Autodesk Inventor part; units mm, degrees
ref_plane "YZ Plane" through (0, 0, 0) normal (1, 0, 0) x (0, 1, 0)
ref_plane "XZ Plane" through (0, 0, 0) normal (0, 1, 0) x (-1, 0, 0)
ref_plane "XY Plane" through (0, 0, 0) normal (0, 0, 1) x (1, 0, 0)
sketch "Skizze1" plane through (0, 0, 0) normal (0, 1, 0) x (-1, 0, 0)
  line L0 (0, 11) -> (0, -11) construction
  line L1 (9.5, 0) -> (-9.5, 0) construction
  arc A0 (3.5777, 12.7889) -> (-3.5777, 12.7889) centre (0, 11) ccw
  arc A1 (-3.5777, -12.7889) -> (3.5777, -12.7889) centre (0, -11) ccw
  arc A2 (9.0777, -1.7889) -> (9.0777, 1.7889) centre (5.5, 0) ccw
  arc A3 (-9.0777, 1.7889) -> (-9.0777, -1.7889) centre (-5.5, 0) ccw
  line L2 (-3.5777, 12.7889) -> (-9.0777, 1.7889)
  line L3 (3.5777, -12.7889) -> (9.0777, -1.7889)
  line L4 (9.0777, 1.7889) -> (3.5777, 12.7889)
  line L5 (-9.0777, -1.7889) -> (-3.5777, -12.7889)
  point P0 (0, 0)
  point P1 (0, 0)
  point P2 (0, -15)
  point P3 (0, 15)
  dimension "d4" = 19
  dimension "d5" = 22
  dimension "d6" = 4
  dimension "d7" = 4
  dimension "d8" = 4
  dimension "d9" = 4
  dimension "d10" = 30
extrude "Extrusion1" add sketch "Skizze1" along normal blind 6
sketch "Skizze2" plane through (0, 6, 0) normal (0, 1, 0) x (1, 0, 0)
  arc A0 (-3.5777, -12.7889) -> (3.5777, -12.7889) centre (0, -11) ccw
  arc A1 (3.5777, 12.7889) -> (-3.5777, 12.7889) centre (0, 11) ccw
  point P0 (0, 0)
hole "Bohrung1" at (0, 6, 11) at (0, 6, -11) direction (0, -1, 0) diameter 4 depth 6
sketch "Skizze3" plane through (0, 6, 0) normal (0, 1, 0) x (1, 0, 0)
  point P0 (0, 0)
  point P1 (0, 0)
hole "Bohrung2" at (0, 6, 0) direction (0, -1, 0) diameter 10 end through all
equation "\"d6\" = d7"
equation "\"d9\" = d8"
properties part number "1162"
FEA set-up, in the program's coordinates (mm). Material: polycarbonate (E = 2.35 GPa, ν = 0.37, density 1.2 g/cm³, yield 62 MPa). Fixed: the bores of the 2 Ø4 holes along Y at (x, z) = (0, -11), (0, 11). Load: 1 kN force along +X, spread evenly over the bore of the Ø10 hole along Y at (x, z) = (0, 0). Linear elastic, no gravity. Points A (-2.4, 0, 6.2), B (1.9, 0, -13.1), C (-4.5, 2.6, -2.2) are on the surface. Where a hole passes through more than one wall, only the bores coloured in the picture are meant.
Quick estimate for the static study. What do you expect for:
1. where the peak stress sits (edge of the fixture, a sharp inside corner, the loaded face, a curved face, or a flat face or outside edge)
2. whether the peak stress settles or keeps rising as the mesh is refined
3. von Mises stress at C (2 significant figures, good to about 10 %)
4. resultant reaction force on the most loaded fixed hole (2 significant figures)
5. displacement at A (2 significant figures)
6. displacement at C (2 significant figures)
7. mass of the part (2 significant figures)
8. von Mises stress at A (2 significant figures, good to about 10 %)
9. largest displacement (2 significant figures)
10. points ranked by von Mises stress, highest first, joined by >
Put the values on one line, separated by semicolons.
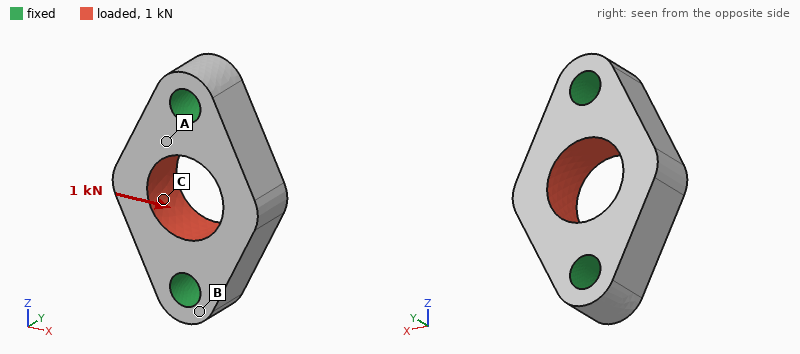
edge of the fixture; keeps rising; 8.9 MPa; 500 N; 43 µm; 77 µm; 1.9 g; 12 MPa; 83 µm; A > C > B
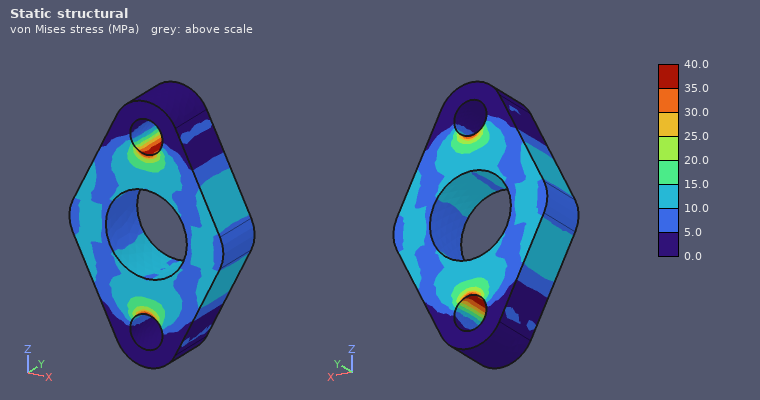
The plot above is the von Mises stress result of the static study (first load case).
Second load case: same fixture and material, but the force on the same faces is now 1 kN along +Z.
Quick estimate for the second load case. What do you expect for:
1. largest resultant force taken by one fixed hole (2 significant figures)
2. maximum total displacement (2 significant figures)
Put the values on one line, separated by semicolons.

500 N; 45 µm
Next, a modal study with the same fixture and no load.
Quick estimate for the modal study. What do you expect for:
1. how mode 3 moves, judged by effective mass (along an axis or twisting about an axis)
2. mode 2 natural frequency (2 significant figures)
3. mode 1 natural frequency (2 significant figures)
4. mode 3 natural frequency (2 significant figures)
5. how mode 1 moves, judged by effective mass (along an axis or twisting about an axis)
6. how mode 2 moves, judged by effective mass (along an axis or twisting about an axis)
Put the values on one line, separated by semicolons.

along X; 11 kHz; 10 kHz; 19 kHz; twisting about Z; along Y
